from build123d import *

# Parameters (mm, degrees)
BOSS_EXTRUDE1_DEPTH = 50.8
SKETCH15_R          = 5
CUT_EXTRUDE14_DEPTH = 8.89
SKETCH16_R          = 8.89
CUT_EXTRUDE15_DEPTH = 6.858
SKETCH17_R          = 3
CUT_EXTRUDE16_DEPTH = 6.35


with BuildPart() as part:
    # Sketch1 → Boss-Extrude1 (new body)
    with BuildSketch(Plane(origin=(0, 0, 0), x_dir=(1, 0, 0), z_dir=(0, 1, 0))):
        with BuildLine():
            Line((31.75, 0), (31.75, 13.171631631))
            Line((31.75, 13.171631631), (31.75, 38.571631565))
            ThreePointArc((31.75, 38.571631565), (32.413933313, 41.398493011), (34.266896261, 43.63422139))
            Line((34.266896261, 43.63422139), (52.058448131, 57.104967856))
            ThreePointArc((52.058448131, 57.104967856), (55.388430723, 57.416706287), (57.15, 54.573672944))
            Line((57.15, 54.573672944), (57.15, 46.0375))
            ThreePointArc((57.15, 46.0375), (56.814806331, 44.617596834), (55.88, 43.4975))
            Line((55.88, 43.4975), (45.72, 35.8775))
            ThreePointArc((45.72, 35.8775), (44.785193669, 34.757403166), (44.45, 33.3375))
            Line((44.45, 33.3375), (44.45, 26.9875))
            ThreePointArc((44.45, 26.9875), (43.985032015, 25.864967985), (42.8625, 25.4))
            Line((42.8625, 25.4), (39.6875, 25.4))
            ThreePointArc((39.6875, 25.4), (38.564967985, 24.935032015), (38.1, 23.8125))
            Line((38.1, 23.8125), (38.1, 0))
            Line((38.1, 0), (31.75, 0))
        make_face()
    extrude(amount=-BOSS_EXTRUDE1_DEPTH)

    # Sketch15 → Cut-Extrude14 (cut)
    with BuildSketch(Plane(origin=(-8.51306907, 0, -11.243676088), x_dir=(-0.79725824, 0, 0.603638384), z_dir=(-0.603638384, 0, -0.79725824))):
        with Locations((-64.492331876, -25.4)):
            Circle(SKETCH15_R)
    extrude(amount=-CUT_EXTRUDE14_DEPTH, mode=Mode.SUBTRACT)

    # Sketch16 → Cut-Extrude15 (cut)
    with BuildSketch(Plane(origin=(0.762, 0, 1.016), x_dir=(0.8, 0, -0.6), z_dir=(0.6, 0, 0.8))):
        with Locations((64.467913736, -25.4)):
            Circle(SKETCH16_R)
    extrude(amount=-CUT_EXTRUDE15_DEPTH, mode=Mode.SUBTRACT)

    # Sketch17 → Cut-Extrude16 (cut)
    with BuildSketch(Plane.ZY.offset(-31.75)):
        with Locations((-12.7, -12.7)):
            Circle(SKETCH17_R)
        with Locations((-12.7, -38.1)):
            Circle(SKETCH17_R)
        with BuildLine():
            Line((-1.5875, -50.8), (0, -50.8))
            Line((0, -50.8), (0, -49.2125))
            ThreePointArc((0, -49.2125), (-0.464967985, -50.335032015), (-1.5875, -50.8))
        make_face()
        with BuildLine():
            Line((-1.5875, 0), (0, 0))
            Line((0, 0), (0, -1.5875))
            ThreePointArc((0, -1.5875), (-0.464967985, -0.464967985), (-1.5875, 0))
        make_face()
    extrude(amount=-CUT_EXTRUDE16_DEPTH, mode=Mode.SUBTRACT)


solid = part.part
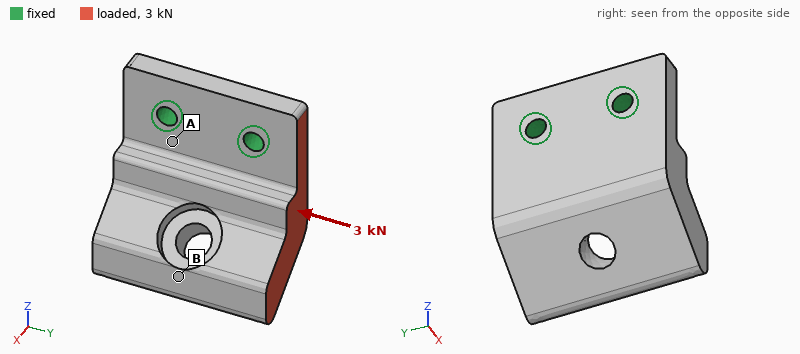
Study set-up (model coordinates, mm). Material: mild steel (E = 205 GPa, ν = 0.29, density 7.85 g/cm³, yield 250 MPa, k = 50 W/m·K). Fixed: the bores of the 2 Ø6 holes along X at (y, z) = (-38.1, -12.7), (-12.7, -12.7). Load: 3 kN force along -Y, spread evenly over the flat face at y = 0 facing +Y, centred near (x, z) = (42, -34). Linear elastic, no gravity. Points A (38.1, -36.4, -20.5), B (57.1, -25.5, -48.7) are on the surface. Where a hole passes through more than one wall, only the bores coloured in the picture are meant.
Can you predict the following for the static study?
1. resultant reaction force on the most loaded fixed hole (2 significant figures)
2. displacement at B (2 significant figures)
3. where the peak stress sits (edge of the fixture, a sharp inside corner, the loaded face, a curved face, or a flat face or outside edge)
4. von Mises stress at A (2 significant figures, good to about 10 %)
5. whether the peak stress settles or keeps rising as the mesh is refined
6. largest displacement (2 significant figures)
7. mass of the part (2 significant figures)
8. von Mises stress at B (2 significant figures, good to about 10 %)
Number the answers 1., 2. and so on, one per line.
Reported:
1. 2.8 kN
2. 11 µm
3. edge of the fixture
4. 34 MPa
5. keeps rising
6. 14 µm
7. 230 g
8. 9.2 MPa
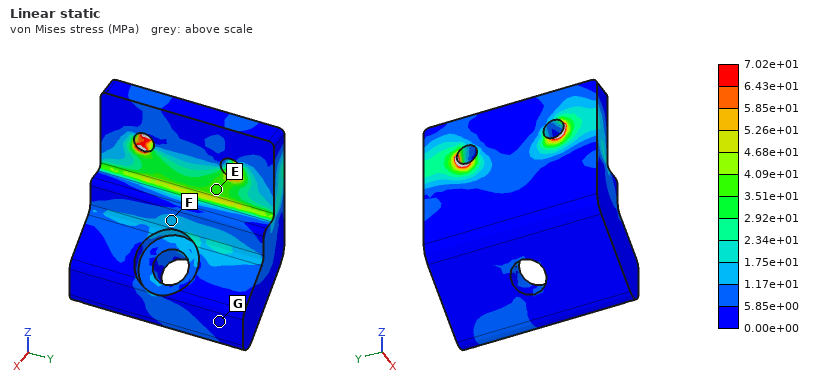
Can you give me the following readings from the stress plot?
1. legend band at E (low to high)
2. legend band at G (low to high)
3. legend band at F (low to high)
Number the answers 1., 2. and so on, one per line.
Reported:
1. 3.51e+01 to 4.09e+01 MPa
2. 0.00e+00 to 5.85e+00 MPa
3. 1.17e+01 to 1.75e+01 MPa
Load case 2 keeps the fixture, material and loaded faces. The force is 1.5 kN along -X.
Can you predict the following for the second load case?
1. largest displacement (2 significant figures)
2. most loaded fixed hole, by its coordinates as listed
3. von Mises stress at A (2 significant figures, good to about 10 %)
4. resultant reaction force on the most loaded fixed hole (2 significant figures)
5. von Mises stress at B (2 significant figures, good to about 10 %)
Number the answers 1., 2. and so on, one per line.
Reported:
1. 85 µm
2. (-12.7, -12.7)
3. 66 MPa
4. 1.9 kN
5. 18 MPa
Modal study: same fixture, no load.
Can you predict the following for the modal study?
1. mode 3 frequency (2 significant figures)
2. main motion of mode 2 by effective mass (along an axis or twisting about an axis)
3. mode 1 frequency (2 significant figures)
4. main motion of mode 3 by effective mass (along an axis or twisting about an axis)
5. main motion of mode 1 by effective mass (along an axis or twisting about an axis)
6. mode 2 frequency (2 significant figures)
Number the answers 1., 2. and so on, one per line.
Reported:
1. 8200 Hz
2. along Y
3. 1900 Hz
4. along Y
5. along X
6. 5000 Hz
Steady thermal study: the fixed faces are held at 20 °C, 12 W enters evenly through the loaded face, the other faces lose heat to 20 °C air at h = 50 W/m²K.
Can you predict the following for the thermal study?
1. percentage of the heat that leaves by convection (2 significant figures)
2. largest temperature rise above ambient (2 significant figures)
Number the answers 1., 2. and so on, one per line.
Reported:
1. 23 %
2. 17 K
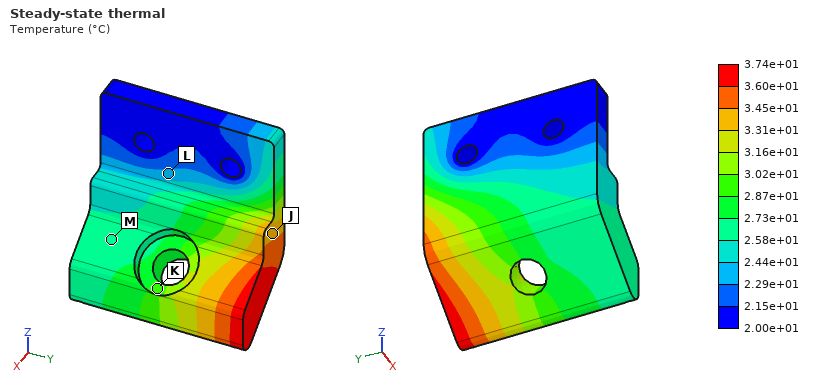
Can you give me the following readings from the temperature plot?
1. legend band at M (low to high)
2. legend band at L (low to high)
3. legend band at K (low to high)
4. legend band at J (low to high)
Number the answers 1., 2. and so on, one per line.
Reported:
1. 2.58e+01 to 2.73e+01 °C
2. 2.29e+01 to 2.44e+01 °C
3. 2.87e+01 to 3.02e+01 °C
4. 3.31e+01 to 3.45e+01 °C
